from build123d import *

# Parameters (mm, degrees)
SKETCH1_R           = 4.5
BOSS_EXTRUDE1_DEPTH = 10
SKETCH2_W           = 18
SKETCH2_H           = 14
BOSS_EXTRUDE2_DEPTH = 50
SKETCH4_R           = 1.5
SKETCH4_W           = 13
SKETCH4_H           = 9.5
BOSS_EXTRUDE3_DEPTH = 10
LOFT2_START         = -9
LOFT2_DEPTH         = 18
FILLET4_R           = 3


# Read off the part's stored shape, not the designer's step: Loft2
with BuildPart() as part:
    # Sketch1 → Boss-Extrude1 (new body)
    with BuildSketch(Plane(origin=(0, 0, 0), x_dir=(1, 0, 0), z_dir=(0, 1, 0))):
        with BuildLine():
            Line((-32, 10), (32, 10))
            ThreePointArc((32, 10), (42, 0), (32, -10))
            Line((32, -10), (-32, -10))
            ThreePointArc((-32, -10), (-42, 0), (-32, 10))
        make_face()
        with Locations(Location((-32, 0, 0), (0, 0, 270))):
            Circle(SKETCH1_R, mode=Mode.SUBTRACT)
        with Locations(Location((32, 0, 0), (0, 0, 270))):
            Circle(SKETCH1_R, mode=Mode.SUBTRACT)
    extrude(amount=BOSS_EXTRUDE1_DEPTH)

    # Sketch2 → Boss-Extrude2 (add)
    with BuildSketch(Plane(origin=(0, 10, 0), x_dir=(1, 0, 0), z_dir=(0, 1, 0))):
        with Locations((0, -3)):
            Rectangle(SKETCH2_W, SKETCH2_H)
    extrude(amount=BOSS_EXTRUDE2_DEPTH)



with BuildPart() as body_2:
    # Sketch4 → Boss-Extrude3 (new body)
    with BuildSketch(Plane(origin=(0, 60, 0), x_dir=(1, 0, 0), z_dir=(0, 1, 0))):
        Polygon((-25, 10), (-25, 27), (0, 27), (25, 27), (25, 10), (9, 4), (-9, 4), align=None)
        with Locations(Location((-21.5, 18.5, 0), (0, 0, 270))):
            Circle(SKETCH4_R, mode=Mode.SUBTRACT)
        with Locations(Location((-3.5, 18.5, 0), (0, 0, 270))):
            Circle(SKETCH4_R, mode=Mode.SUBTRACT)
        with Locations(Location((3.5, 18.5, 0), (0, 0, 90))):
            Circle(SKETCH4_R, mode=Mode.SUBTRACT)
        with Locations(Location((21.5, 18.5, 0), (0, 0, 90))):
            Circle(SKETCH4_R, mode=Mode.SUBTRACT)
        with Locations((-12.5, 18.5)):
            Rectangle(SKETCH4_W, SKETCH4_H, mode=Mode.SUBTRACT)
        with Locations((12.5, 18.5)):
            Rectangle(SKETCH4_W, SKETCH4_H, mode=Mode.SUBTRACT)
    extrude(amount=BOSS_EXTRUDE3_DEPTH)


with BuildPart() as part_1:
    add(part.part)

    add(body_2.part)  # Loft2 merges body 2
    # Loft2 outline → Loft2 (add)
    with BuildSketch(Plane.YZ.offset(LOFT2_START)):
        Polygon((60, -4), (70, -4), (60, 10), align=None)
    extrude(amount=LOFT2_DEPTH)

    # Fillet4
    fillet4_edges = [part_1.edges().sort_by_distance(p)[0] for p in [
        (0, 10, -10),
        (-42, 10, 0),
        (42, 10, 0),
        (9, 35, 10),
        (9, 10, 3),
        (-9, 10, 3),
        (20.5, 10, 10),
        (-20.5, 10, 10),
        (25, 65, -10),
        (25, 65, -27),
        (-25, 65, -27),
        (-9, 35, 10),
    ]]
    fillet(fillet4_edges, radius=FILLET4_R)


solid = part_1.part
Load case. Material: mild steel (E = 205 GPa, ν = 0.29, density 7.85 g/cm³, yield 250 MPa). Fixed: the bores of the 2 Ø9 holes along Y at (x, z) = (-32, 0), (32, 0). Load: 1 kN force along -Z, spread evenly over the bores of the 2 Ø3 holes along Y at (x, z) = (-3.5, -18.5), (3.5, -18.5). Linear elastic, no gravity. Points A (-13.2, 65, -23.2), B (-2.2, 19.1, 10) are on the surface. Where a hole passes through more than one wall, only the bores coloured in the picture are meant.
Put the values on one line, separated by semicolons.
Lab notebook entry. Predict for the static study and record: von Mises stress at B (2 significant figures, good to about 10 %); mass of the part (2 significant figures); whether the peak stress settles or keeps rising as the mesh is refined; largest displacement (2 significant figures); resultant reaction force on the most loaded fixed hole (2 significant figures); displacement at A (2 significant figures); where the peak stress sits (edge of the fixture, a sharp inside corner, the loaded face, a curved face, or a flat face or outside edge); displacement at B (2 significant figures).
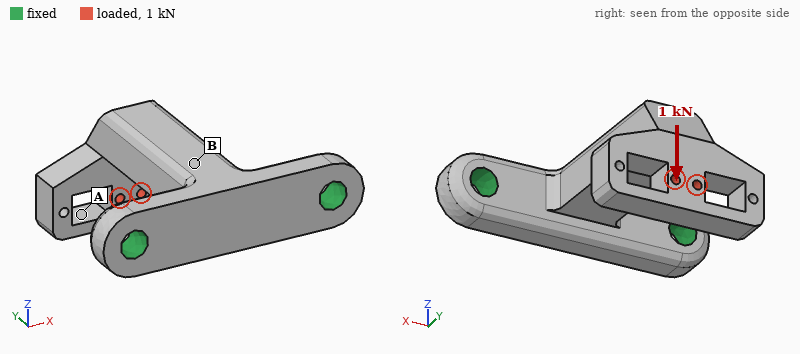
79 MPa; 280 g; keeps rising; 0.23 mm; 510 N; 0.21 mm; a sharp inside corner; 0.039 mm
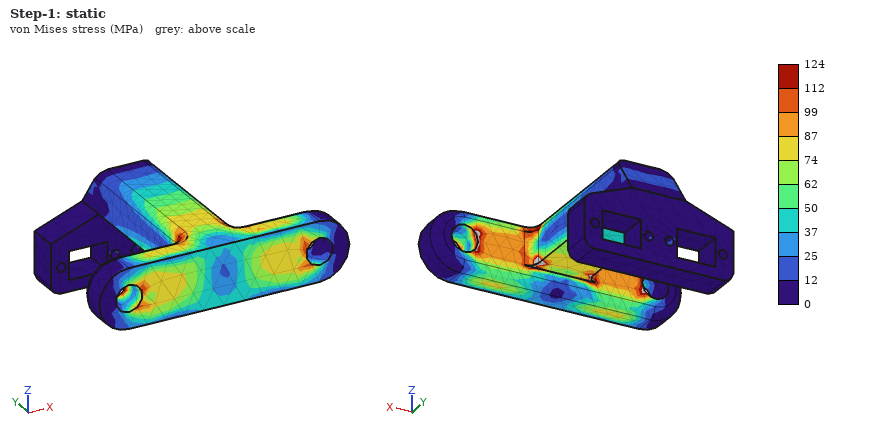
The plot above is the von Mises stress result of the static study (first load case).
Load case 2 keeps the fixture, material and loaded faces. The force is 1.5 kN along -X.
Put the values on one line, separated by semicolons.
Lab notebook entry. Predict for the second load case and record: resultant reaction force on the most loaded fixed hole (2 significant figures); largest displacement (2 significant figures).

2.3 kN; 0.22 mm
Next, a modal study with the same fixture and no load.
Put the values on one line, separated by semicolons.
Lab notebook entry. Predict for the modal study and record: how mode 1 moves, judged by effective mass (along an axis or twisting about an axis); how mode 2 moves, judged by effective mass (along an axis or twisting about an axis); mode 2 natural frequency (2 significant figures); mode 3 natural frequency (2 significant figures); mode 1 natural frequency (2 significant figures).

along Z; along X; 1700 Hz; 3600 Hz; 1100 Hz
